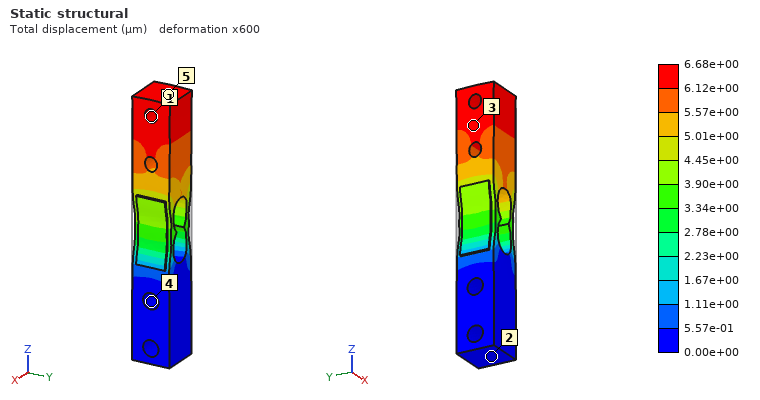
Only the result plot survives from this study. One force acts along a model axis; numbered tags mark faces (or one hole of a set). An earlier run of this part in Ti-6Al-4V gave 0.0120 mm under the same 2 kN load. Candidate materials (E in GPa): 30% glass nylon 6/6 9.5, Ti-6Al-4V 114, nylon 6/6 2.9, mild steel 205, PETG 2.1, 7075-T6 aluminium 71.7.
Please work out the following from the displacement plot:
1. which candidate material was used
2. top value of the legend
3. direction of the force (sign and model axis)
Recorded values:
mild steel
6.68e+00 µm
+Z
